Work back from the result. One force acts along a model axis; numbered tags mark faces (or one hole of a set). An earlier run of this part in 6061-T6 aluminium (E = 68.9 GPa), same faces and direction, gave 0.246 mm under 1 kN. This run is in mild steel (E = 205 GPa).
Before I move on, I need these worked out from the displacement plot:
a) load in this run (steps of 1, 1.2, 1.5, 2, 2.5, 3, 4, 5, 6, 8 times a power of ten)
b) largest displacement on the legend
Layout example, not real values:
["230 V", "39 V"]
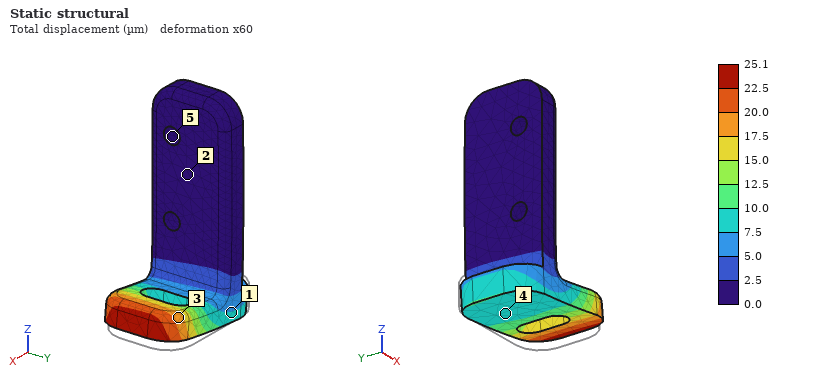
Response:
["300 N", "25.1 µm"]
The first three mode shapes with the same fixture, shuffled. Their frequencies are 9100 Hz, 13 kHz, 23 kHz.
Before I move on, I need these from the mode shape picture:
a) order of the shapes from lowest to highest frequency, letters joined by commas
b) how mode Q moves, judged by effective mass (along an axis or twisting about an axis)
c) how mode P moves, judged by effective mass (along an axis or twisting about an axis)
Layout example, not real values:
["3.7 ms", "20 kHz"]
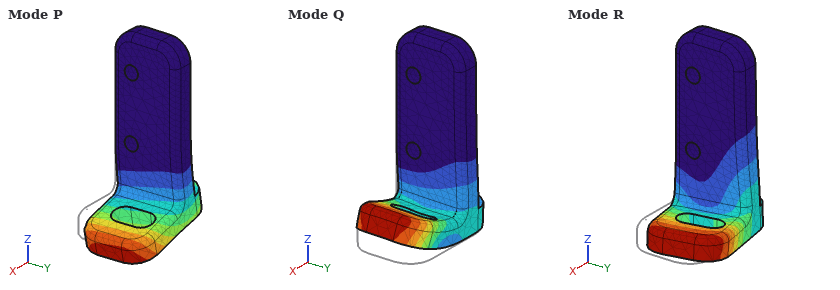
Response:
["P, R, Q", "along X", "along X"]
